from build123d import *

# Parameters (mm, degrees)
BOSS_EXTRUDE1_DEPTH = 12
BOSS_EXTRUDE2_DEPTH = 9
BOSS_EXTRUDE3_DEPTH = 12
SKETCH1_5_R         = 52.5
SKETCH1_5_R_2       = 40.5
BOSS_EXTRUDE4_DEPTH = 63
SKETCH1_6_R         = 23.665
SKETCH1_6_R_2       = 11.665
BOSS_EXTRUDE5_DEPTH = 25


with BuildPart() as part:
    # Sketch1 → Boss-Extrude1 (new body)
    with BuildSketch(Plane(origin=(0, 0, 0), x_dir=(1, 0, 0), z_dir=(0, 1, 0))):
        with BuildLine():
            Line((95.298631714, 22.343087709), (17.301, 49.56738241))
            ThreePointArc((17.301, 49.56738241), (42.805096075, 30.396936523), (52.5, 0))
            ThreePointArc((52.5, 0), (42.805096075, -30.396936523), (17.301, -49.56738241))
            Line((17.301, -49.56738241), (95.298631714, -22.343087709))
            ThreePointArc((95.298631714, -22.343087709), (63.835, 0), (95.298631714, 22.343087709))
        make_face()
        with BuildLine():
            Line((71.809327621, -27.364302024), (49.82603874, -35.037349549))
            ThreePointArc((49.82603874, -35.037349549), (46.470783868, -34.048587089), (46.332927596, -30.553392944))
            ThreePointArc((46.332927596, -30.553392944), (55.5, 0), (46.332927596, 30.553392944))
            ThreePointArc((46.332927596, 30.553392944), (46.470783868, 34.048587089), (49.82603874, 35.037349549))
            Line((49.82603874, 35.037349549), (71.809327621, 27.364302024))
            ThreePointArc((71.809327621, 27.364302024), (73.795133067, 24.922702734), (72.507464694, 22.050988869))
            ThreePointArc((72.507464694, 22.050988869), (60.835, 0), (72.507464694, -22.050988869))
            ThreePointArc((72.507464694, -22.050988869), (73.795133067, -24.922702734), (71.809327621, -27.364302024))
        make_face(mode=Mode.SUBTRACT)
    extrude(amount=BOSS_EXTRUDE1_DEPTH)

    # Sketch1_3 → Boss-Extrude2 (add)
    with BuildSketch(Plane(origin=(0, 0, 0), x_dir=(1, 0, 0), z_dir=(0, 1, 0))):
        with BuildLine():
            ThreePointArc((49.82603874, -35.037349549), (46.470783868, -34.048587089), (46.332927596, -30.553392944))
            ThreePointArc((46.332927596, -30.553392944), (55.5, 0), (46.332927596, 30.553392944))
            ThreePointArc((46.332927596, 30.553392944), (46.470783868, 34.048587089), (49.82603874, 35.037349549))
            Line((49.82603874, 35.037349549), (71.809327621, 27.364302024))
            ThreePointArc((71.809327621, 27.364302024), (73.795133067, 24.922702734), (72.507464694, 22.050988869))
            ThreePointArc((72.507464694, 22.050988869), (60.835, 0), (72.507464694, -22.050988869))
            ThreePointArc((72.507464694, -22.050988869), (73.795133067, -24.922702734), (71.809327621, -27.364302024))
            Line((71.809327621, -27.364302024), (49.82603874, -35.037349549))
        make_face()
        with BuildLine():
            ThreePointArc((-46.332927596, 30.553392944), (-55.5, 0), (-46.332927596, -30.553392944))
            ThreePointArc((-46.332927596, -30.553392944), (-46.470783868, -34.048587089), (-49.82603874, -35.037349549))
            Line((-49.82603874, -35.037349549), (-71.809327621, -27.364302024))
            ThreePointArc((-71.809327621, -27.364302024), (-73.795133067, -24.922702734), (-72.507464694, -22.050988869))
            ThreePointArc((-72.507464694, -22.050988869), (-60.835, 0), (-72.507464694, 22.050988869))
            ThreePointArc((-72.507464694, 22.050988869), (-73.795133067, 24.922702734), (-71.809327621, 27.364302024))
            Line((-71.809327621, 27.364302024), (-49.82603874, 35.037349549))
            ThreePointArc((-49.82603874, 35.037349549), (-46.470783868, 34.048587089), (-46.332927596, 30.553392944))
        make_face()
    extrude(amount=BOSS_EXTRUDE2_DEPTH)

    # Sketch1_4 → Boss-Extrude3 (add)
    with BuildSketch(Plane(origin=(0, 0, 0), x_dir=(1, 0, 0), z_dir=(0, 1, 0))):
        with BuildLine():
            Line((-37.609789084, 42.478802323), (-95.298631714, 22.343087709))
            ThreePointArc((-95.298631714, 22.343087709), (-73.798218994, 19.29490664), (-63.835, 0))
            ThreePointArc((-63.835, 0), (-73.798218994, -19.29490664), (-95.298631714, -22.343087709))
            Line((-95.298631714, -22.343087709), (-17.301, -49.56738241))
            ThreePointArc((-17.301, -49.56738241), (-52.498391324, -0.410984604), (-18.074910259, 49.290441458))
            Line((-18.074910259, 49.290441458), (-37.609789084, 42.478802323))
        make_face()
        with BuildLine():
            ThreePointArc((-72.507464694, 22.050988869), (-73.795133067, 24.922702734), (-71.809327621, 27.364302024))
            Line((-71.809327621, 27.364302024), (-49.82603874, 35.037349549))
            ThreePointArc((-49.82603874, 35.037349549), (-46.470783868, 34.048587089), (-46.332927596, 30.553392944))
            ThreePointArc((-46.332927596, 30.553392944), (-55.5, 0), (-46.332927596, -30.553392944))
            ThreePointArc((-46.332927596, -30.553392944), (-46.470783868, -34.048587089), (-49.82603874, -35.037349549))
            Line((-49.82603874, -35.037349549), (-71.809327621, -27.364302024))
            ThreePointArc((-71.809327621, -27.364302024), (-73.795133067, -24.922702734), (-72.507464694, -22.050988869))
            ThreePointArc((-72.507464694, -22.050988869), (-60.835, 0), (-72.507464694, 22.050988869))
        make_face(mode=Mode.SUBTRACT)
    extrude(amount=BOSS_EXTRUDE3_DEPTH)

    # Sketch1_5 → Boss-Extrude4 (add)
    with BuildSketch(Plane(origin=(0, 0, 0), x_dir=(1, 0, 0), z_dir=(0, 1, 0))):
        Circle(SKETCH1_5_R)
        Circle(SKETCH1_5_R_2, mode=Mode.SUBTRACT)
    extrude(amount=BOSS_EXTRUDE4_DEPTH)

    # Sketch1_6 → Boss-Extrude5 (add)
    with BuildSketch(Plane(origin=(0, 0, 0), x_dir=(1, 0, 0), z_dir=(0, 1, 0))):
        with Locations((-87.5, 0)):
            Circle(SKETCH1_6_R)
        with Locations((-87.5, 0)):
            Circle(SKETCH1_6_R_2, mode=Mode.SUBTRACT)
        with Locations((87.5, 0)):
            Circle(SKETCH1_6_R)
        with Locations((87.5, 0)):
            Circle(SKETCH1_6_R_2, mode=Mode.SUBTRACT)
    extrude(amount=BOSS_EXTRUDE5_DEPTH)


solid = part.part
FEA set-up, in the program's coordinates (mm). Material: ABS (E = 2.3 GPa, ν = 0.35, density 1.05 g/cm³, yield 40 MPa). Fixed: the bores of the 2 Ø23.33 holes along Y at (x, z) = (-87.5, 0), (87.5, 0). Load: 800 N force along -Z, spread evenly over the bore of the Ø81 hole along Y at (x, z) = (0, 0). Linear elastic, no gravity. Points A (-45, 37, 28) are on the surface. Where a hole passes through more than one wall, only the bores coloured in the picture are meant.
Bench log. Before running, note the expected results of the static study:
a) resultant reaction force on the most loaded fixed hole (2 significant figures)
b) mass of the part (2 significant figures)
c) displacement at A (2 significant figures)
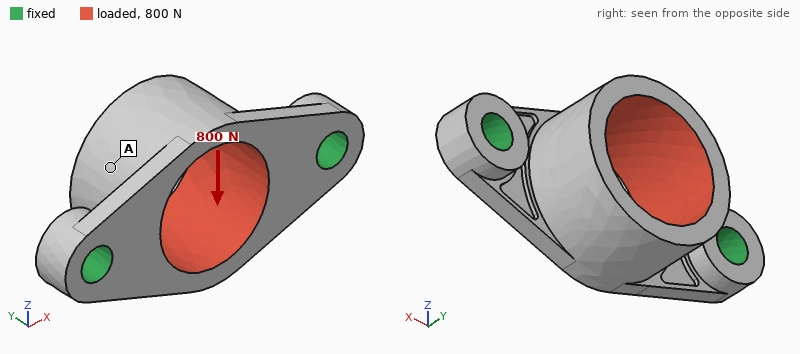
400 N
340 g
0.36 mm
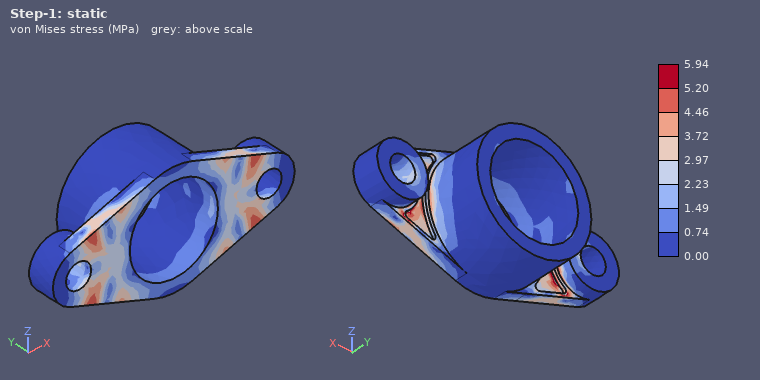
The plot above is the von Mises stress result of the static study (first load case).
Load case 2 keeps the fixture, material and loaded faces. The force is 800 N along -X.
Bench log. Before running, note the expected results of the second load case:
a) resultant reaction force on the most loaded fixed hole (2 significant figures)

440 N
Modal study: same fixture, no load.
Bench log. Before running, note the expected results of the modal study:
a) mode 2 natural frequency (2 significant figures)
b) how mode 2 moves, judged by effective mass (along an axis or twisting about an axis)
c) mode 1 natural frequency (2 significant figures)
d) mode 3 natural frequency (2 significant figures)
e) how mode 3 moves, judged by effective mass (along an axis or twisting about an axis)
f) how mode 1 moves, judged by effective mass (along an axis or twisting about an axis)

770 Hz
along Y
360 Hz
1200 Hz
along X
along Z
